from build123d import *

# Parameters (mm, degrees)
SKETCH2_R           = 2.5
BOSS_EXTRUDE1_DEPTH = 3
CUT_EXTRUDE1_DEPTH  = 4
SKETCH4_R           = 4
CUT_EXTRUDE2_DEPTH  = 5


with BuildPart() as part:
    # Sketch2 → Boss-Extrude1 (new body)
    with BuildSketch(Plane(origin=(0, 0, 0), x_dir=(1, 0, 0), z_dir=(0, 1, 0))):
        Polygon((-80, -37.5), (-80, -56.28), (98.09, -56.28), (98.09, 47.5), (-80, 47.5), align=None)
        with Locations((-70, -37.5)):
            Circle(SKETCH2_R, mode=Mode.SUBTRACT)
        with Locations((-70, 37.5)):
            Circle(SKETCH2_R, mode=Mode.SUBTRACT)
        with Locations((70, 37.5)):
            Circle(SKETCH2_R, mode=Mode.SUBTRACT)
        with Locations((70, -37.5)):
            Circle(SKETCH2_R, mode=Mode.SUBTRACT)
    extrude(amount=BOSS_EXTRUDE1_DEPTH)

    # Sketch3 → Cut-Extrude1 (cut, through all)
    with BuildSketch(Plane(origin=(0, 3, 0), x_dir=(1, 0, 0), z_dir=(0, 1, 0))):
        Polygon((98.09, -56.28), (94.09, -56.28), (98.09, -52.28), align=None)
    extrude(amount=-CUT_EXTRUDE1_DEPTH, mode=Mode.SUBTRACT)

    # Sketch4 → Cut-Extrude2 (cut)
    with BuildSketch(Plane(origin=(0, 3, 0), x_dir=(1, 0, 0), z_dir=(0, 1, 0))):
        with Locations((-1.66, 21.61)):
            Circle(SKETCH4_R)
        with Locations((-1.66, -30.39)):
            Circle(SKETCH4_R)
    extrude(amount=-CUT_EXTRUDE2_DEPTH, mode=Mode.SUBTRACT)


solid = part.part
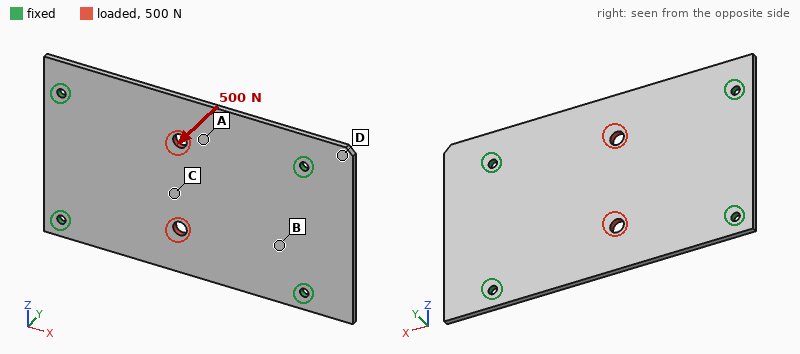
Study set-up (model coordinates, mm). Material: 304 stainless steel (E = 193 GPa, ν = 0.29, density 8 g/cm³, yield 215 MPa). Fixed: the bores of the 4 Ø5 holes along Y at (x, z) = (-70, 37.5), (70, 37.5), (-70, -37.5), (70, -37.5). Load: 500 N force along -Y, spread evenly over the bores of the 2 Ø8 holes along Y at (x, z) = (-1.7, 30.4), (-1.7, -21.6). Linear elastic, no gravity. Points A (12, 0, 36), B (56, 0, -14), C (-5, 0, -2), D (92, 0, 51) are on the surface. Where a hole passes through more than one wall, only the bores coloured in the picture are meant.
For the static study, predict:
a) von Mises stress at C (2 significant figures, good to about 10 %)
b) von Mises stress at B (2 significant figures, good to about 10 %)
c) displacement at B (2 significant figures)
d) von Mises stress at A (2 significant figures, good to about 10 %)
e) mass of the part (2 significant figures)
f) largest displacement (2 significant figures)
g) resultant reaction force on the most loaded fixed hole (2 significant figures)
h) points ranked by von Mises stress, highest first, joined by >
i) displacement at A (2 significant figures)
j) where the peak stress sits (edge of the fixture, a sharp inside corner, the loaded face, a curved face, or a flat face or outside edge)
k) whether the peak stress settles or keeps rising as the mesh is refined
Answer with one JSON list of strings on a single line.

["49 MPa", "23 MPa", "0.038 mm", "32 MPa", "440 g", "0.20 mm", "140 N", "C > A > B > D", "0.17 mm", "edge of the fixture", "keeps rising"]
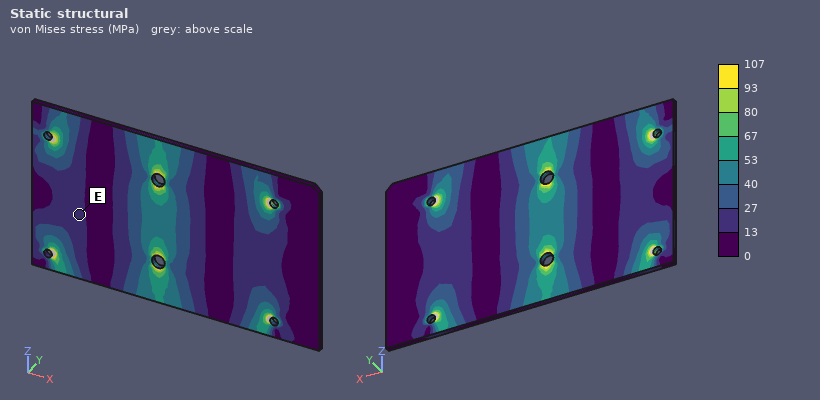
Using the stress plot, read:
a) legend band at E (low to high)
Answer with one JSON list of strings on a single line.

["13 to 27 MPa"]
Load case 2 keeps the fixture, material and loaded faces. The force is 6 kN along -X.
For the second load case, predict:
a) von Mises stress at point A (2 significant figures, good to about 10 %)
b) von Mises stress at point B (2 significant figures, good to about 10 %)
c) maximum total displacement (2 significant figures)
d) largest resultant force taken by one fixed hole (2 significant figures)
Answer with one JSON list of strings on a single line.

["19 MPa", "6.8 MPa", "6.6 µm", "1.7 kN"]
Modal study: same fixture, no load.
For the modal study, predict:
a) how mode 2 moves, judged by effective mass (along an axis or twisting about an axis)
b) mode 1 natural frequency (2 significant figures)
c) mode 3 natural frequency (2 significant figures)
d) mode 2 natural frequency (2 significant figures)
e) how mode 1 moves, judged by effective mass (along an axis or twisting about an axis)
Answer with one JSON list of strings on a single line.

["twisting about X", "690 Hz", "1800 Hz", "1000 Hz", "along Y"]
